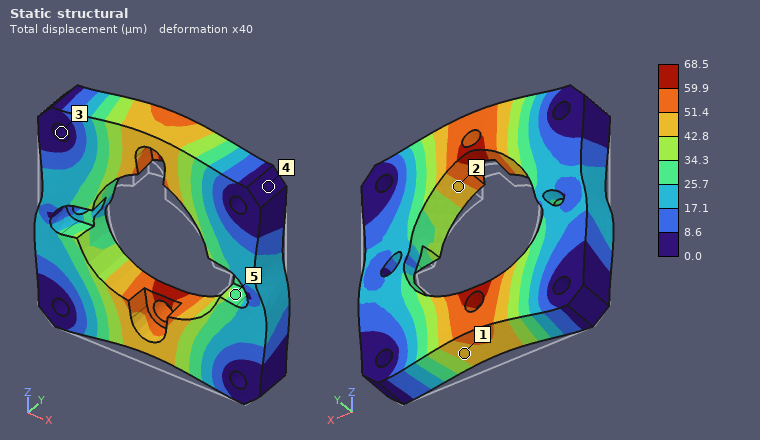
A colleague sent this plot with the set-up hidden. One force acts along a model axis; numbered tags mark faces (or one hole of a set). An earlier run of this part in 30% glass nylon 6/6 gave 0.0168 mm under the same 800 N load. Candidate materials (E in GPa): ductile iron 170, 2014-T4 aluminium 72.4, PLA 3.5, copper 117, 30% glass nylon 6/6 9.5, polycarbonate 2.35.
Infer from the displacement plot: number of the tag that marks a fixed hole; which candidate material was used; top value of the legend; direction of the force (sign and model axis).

3
polycarbonate
68.5 µm
+Z
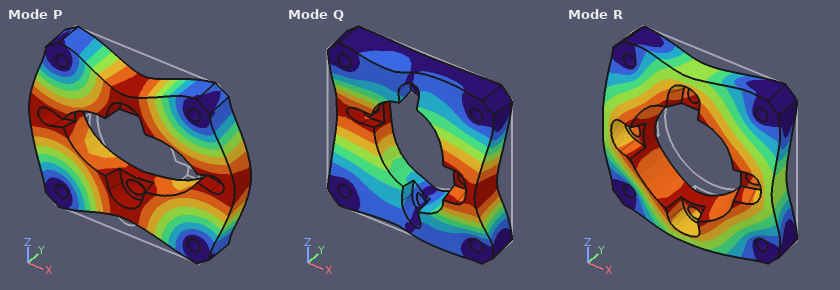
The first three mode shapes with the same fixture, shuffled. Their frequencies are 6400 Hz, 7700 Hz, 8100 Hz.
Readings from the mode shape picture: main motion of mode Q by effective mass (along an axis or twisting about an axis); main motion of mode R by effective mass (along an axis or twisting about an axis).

twisting about Z
along Y
